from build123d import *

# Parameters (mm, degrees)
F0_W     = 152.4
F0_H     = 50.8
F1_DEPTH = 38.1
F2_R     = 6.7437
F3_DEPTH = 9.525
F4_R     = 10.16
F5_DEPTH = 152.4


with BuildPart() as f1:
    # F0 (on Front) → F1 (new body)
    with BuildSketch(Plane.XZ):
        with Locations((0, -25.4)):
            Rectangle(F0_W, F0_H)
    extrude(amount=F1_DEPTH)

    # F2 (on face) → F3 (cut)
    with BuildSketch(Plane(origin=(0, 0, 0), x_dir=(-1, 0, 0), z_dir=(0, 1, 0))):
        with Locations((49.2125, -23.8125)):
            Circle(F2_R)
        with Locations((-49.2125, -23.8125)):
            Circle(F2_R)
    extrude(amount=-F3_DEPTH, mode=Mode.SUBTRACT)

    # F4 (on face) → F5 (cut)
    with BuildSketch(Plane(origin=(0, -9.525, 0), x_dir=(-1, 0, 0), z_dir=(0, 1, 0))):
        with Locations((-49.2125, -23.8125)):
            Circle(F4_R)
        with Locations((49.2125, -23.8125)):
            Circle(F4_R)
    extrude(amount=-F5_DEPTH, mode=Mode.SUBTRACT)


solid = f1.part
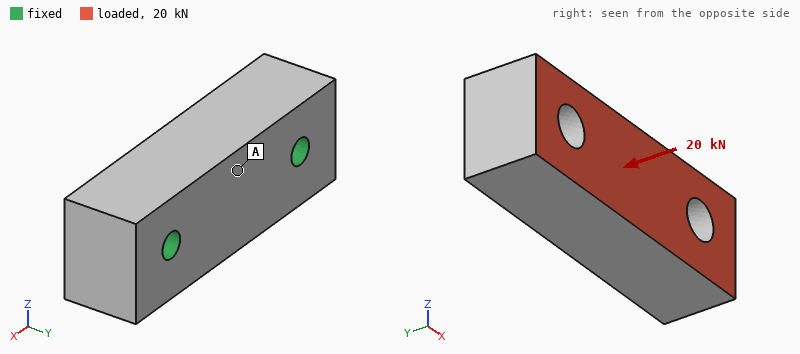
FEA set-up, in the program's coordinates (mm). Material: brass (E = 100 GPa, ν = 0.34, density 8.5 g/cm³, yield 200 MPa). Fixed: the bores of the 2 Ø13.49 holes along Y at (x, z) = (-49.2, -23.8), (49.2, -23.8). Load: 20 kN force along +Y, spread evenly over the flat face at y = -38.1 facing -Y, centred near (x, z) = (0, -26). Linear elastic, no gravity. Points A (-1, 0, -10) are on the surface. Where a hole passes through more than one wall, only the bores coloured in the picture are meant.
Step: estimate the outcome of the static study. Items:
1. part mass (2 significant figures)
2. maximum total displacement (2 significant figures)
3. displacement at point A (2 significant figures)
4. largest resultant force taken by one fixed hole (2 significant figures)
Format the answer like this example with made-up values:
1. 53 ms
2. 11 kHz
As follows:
1. 2.3 kg
2. 14 µm
3. 7.4 µm
4. 10 kN
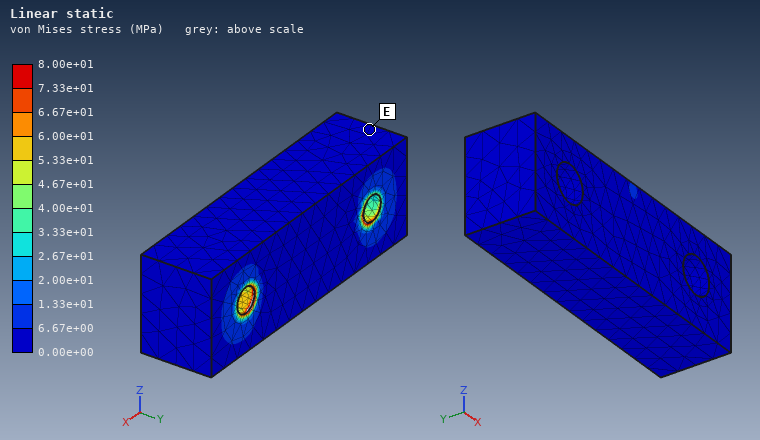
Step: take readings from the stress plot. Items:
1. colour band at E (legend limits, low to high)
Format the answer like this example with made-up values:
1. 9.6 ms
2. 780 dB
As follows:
1. 0.00e+00 to 6.67e+00 MPa
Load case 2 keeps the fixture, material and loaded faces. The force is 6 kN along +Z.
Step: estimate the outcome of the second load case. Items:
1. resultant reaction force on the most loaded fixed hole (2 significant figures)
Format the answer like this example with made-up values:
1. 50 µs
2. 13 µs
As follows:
1. 3.0 kN
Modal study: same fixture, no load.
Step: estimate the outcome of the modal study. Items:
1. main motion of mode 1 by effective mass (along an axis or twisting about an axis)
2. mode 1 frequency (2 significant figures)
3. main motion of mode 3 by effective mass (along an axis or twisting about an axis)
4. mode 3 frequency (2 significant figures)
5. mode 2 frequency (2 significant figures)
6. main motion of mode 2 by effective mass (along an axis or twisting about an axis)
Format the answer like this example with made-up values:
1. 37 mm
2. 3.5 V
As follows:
1. along Z
2. 2300 Hz
3. along Y
4. 5200 Hz
5. 4900 Hz
6. twisting about Y
